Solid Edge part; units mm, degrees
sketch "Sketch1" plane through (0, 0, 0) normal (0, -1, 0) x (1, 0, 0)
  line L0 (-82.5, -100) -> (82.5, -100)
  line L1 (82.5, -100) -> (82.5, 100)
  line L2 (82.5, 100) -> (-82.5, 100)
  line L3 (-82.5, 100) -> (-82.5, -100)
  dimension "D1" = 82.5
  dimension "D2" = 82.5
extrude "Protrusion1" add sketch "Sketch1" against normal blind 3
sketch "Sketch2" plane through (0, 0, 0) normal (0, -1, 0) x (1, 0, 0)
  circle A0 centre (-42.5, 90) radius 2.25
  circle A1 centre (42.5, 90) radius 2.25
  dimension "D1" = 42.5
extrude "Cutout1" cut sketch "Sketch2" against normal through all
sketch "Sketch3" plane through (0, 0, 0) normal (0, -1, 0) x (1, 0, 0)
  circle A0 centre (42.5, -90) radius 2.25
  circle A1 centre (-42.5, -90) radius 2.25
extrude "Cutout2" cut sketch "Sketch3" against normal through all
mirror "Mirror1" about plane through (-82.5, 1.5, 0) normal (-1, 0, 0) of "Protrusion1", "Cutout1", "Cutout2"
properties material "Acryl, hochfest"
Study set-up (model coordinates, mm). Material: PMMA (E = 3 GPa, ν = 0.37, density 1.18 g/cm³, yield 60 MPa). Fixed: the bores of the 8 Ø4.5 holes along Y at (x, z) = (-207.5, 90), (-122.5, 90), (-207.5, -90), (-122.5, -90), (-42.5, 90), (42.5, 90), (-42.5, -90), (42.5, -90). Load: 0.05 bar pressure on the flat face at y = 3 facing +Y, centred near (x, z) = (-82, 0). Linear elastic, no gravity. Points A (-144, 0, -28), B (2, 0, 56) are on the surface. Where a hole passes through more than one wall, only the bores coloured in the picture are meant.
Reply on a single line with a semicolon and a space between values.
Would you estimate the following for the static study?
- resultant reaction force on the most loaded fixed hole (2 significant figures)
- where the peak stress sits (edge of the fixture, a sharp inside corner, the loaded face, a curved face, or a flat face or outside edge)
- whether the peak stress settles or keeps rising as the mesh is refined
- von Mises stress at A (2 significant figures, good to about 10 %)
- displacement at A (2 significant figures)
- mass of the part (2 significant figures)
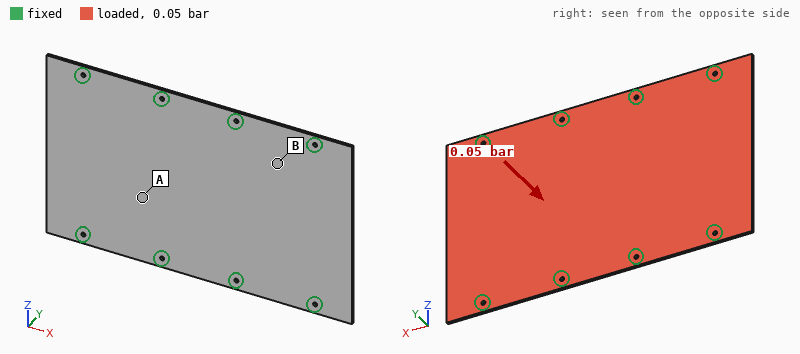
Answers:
43 N; edge of the fixture; keeps rising; 3.6 MPa; 2.2 mm; 230 g
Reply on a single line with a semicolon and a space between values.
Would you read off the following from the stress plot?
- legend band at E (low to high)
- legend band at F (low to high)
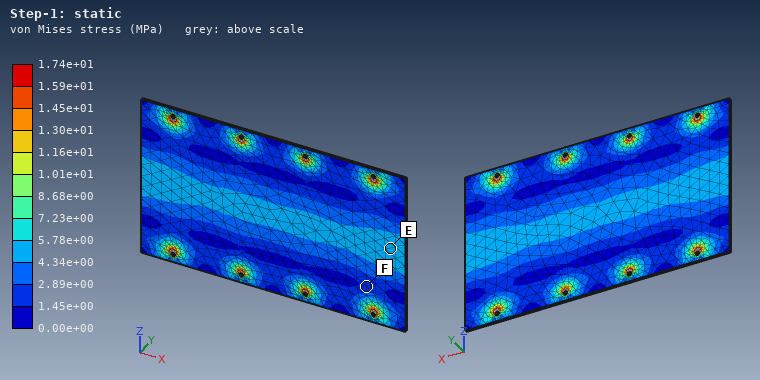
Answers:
4.34e+00 to 5.78e+00 MPa; 1.45e+00 to 2.89e+00 MPa
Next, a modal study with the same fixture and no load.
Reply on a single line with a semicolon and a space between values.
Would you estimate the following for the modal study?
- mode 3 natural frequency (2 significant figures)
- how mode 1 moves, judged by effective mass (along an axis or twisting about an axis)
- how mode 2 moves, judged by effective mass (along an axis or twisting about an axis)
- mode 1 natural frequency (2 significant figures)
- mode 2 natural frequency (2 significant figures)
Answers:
170 Hz; along Y; twisting about Z; 130 Hz; 140 Hz
